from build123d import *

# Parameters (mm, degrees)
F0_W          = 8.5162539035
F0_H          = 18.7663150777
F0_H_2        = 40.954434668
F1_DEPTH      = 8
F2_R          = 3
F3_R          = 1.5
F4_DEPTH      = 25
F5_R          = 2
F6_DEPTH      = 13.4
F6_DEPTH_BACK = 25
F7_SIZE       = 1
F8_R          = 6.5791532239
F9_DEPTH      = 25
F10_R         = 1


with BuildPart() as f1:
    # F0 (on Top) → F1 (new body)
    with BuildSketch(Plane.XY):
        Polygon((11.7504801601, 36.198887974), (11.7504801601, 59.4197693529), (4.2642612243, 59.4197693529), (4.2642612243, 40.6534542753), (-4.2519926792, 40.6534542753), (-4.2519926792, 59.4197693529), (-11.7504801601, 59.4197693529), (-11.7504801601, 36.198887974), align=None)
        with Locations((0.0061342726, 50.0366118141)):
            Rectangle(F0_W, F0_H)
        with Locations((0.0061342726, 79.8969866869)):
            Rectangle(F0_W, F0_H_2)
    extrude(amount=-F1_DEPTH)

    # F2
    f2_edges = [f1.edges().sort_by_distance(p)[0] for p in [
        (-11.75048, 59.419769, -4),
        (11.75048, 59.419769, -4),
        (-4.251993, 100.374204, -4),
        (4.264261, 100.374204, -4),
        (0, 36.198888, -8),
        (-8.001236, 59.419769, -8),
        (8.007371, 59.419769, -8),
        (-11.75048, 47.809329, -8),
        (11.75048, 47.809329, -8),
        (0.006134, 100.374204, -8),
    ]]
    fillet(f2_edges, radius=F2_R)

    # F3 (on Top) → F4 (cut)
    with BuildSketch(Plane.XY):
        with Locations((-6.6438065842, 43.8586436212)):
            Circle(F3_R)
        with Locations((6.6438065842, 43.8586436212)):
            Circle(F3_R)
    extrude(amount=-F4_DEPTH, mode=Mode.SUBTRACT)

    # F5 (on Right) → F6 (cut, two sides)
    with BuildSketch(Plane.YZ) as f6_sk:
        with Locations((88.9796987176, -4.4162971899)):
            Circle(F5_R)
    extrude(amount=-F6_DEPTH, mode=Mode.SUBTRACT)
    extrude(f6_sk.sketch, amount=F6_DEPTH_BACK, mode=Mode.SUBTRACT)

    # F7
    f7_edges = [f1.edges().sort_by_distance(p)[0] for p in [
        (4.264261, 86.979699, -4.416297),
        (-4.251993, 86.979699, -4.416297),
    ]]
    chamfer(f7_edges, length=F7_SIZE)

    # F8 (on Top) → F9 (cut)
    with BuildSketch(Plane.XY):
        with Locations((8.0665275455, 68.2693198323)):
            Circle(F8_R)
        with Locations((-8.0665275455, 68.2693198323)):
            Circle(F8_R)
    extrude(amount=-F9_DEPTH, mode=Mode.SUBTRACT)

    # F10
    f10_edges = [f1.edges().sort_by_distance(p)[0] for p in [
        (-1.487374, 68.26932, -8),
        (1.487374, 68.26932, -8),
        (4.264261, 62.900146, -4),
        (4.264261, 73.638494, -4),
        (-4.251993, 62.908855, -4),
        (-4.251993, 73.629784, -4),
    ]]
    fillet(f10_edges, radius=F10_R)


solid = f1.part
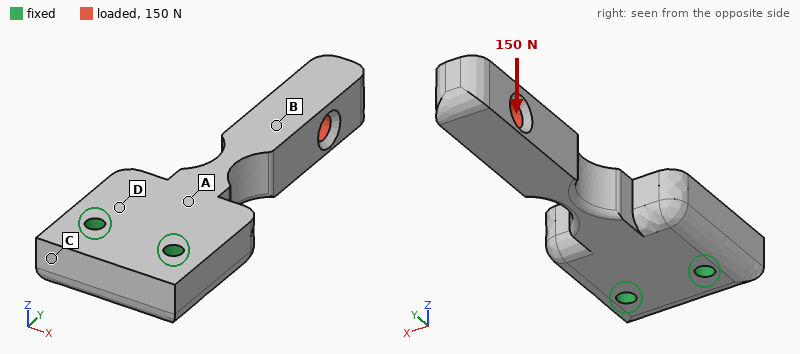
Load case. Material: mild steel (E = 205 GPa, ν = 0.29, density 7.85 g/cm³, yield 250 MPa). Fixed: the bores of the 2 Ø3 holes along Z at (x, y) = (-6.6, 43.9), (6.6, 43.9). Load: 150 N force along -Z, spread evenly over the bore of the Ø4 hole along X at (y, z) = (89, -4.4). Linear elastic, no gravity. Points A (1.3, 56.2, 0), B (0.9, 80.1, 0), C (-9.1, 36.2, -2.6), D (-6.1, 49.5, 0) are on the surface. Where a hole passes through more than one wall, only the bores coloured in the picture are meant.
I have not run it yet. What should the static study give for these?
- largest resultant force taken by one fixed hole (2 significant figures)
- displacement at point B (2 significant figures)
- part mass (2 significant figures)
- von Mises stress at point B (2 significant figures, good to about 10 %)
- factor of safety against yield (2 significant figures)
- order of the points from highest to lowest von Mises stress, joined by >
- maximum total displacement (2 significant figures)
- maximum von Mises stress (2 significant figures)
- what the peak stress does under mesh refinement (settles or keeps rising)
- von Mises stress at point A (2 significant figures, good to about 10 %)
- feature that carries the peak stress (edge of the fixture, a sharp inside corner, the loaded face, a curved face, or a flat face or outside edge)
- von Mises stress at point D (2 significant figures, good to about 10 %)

75 N
37 µm
50 g
15 MPa
2.3
A > D > B > C
80 µm
110 MPa
settles
40 MPa
a curved face
26 MPa
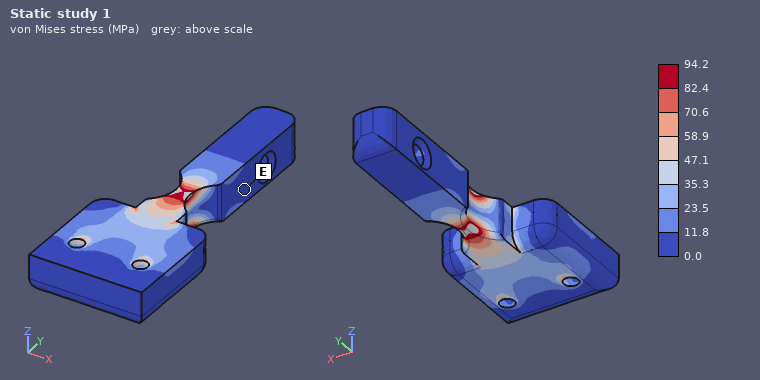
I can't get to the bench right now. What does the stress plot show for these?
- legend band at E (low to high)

0.0 to 11.8 MPa
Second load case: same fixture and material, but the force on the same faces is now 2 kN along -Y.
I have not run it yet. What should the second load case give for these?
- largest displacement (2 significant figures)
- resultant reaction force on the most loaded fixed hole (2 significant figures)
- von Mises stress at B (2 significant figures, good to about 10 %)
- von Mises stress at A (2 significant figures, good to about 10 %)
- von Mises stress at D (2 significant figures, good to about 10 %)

23 µm
1.0 kN
22 MPa
15 MPa
12 MPa
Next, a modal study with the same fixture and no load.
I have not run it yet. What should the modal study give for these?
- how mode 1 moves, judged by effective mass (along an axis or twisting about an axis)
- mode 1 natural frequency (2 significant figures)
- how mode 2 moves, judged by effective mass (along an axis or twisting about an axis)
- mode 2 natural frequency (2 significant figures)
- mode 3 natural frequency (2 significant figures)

along X
1600 Hz
along Z
2400 Hz
11 kHz
